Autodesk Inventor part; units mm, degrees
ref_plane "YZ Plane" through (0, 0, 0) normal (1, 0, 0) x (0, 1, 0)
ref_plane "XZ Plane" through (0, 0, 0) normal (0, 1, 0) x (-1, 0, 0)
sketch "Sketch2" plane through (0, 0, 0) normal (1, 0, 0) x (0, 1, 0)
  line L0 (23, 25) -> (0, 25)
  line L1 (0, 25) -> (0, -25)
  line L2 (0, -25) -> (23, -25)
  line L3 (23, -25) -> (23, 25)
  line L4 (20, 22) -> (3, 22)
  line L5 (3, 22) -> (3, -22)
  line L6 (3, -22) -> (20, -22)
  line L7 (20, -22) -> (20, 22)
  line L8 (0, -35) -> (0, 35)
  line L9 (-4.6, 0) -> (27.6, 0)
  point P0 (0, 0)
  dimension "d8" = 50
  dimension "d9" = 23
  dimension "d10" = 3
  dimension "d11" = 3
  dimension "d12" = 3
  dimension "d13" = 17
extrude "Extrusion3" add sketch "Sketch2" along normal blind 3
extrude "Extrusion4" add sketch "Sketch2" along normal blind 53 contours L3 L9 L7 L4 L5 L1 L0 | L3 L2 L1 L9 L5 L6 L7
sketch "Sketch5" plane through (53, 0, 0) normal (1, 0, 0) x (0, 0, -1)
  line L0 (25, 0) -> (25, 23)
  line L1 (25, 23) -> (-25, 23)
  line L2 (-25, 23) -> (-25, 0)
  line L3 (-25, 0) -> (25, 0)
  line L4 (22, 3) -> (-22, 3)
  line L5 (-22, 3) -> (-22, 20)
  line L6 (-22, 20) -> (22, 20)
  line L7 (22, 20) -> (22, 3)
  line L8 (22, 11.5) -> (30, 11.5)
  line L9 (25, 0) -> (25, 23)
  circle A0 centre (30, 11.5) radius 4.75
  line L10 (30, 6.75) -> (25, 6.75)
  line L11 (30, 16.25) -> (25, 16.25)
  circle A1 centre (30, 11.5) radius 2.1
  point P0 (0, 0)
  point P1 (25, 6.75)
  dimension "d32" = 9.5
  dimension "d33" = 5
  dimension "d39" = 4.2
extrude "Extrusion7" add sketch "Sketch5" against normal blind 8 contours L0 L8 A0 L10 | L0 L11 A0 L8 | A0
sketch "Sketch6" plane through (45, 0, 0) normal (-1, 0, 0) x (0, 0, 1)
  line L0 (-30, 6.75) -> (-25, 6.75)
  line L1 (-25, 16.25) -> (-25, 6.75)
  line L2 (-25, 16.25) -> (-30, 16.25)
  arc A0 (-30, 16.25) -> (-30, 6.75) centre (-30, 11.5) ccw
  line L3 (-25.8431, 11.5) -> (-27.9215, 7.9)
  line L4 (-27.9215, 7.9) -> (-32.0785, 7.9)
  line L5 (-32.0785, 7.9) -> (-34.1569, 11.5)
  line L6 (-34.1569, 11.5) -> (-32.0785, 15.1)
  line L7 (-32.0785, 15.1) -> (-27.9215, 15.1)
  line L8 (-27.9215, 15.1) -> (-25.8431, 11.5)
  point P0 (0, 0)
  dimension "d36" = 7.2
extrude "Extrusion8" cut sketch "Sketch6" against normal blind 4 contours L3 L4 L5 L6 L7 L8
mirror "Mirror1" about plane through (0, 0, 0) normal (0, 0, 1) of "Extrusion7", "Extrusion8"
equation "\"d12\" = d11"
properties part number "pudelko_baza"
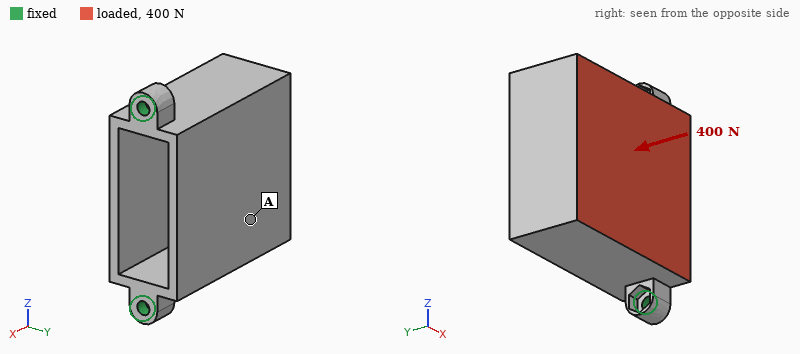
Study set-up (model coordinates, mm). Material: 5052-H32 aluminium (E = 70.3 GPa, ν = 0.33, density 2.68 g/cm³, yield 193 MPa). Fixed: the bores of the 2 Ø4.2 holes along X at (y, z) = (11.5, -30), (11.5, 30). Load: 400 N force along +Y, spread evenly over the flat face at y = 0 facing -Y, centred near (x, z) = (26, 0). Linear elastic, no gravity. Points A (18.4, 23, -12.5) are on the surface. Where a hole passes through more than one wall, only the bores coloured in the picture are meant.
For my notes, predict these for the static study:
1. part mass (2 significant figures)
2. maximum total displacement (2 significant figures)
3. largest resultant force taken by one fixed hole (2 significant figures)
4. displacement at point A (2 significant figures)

65 g
0.16 mm
210 N
0.10 mm
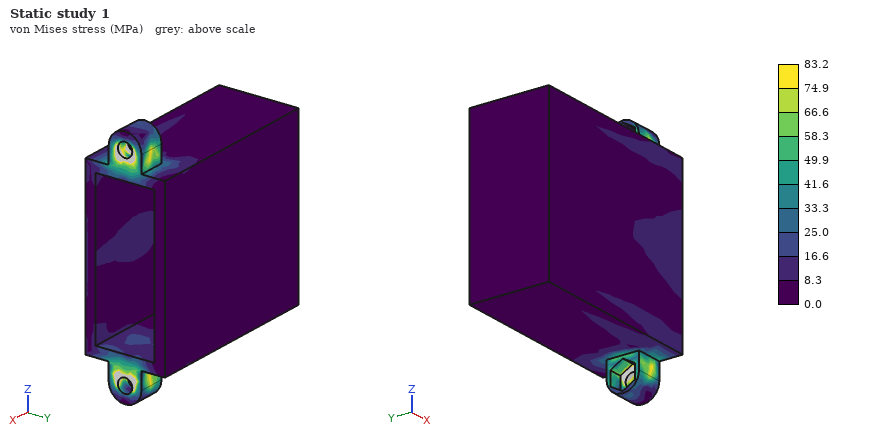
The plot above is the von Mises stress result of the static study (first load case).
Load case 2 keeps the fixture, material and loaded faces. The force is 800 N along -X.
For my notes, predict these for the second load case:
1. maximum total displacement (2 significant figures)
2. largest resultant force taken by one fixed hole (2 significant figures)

0.15 mm
420 N
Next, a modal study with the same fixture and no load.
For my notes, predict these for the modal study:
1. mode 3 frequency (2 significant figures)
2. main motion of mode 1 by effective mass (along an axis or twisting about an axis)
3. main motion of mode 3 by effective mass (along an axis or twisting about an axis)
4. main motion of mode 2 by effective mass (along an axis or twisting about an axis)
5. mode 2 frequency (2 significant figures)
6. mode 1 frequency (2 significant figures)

5700 Hz
along Y
twisting about X
along Z
5200 Hz
1100 Hz
